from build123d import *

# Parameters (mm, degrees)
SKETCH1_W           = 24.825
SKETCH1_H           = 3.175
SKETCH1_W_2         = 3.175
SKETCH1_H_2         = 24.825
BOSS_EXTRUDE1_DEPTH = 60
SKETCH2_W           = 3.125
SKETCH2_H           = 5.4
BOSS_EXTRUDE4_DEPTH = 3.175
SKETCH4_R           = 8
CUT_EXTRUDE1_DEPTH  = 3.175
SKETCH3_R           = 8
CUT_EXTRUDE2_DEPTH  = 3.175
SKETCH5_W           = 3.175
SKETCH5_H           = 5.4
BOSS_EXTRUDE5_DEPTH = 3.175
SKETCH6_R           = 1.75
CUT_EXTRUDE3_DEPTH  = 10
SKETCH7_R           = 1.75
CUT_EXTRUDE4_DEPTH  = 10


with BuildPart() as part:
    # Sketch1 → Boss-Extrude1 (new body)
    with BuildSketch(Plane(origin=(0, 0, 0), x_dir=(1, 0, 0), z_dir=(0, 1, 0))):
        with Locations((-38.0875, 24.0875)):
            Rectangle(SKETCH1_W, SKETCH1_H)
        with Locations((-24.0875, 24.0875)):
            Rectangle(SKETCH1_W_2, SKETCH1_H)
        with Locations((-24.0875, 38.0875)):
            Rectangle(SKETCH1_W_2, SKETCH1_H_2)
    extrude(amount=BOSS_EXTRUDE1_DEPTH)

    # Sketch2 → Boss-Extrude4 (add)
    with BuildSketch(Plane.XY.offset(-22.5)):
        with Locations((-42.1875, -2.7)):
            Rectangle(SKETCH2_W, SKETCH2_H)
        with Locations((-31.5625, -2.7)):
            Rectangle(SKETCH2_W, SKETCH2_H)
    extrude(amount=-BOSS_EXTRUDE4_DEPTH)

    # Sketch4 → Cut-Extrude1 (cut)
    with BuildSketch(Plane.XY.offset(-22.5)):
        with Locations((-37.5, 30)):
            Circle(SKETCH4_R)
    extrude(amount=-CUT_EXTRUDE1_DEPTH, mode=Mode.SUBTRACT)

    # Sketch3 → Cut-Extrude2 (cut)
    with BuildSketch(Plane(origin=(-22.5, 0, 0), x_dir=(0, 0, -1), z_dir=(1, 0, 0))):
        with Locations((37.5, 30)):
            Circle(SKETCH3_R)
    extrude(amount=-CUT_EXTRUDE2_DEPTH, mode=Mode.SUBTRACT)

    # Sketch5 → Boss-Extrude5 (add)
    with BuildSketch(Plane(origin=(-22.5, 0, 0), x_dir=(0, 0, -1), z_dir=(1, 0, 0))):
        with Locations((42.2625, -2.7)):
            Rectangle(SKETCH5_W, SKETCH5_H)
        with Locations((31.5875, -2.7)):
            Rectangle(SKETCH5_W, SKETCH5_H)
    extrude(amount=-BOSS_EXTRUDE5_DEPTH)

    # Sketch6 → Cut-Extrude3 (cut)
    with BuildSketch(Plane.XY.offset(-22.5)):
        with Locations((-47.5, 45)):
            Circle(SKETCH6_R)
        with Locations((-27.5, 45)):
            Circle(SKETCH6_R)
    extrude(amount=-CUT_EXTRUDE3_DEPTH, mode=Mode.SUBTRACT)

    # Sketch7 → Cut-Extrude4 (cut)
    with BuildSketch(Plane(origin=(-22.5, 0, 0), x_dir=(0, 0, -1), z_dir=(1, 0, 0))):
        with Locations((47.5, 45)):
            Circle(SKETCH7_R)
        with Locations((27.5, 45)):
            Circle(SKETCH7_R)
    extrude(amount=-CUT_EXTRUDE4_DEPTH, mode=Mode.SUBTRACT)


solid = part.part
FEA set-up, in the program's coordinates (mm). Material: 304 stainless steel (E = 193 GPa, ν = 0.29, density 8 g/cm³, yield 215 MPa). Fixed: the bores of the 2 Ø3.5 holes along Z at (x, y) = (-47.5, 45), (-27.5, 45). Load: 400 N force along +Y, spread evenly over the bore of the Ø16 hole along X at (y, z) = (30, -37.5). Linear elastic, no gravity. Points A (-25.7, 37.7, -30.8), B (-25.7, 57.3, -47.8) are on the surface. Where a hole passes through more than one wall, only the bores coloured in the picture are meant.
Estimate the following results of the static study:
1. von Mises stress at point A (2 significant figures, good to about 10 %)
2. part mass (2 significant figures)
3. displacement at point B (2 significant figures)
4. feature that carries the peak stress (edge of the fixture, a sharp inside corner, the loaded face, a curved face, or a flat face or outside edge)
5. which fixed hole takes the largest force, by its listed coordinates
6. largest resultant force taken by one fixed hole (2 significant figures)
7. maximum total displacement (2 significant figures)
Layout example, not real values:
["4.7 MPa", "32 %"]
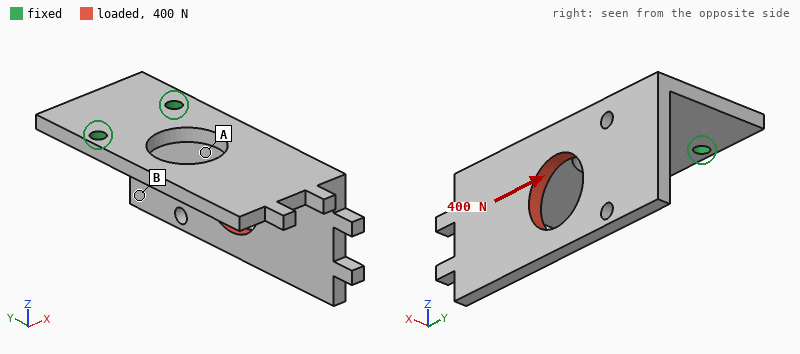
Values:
["23 MPa", "71 g", "31 µm", "edge of the fixture", "(-27.5, 45)", "440 N", "64 µm"]
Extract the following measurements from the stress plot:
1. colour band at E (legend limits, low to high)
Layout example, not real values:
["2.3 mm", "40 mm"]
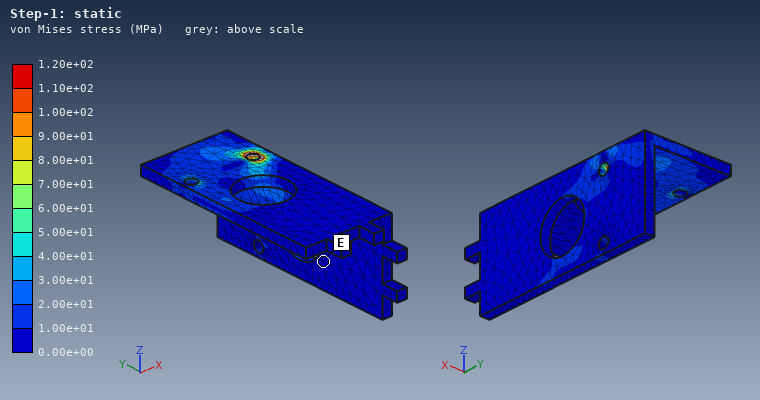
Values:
["0.00e+00 to 1.00e+01 MPa"]
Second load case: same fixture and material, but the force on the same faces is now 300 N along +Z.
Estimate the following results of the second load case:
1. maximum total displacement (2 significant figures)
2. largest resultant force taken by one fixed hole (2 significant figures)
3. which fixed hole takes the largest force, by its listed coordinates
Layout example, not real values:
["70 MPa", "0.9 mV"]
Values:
["57 µm", "310 N", "(-27.5, 45)"]
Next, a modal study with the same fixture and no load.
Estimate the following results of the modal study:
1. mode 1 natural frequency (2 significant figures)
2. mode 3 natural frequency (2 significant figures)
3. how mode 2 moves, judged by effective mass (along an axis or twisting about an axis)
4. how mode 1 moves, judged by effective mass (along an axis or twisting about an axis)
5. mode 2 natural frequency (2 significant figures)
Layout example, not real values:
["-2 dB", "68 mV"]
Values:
["1500 Hz", "3500 Hz", "along X", "along Z", "1900 Hz"]
